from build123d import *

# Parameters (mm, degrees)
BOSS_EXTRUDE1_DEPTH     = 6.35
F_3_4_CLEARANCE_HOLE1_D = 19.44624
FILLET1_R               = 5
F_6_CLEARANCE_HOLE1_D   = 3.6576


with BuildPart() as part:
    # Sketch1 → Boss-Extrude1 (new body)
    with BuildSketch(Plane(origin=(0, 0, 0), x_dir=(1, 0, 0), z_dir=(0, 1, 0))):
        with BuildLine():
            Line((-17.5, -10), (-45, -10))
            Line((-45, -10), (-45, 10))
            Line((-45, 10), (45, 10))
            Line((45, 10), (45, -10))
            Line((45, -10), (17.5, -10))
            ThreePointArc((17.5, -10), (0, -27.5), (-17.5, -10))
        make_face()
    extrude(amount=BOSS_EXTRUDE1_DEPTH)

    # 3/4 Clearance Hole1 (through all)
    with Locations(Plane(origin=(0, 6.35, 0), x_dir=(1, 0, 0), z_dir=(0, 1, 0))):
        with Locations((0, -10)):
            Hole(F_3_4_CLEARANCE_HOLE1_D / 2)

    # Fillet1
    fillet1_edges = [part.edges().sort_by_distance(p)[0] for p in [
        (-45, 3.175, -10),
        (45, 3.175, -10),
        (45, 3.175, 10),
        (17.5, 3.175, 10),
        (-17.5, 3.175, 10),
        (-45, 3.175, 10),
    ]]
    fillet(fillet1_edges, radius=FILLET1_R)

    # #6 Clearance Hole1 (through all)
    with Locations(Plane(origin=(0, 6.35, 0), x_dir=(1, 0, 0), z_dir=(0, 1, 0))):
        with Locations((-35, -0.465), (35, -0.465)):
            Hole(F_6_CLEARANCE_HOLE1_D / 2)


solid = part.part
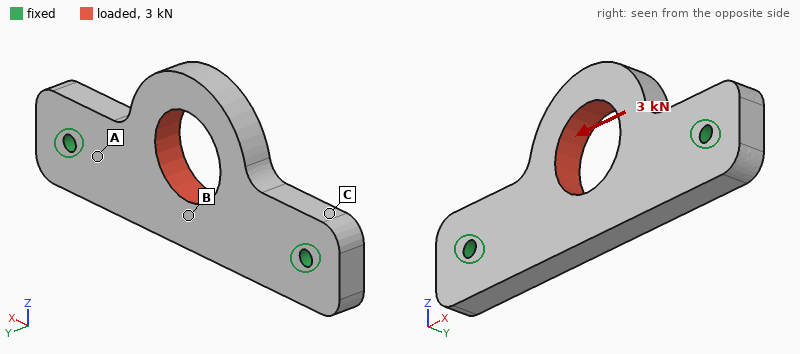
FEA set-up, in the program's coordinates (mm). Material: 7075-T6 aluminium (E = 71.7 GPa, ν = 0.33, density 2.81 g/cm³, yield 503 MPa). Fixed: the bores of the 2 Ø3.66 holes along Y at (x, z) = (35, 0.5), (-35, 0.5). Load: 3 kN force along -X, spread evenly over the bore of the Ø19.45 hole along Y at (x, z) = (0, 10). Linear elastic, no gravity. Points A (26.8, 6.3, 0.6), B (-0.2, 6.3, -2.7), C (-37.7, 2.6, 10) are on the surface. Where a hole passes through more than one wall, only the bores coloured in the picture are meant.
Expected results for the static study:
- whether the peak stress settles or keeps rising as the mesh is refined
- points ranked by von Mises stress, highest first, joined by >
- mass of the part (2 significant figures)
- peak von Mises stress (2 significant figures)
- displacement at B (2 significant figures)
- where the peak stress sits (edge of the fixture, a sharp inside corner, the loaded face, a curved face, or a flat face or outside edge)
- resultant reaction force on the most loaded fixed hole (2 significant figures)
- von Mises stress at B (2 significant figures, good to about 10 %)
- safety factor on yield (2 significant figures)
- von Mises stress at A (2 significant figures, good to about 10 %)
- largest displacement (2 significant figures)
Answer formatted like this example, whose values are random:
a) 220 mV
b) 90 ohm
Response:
a) settles
b) A > B > C
c) 35 g
d) 62 MPa
e) 4.0 µm
f) a curved face
g) 1.6 kN
h) 9.4 MPa
i) 8.2
j) 17 MPa
k) 18 µm
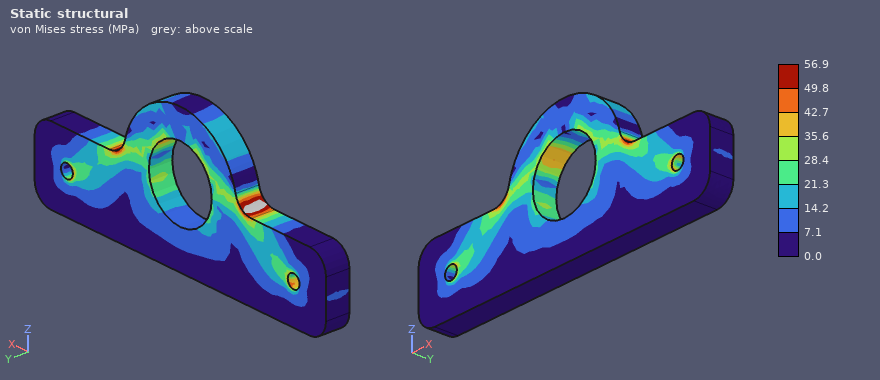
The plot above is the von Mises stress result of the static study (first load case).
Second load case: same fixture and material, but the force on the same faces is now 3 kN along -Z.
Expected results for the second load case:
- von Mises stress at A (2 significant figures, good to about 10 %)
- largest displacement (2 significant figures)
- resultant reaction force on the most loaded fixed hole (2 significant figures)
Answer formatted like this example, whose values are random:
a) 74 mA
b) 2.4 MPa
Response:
a) 31 MPa
b) 49 µm
c) 1.6 kN
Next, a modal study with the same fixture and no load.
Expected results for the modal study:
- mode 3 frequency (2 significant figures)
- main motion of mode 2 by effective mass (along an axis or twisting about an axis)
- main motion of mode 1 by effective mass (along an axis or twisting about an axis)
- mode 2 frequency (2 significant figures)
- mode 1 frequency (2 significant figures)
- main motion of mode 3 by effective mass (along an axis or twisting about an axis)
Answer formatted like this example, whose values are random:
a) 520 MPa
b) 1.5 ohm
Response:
a) 9900 Hz
b) along Y
c) along Y
d) 7000 Hz
e) 4300 Hz
f) along Z
